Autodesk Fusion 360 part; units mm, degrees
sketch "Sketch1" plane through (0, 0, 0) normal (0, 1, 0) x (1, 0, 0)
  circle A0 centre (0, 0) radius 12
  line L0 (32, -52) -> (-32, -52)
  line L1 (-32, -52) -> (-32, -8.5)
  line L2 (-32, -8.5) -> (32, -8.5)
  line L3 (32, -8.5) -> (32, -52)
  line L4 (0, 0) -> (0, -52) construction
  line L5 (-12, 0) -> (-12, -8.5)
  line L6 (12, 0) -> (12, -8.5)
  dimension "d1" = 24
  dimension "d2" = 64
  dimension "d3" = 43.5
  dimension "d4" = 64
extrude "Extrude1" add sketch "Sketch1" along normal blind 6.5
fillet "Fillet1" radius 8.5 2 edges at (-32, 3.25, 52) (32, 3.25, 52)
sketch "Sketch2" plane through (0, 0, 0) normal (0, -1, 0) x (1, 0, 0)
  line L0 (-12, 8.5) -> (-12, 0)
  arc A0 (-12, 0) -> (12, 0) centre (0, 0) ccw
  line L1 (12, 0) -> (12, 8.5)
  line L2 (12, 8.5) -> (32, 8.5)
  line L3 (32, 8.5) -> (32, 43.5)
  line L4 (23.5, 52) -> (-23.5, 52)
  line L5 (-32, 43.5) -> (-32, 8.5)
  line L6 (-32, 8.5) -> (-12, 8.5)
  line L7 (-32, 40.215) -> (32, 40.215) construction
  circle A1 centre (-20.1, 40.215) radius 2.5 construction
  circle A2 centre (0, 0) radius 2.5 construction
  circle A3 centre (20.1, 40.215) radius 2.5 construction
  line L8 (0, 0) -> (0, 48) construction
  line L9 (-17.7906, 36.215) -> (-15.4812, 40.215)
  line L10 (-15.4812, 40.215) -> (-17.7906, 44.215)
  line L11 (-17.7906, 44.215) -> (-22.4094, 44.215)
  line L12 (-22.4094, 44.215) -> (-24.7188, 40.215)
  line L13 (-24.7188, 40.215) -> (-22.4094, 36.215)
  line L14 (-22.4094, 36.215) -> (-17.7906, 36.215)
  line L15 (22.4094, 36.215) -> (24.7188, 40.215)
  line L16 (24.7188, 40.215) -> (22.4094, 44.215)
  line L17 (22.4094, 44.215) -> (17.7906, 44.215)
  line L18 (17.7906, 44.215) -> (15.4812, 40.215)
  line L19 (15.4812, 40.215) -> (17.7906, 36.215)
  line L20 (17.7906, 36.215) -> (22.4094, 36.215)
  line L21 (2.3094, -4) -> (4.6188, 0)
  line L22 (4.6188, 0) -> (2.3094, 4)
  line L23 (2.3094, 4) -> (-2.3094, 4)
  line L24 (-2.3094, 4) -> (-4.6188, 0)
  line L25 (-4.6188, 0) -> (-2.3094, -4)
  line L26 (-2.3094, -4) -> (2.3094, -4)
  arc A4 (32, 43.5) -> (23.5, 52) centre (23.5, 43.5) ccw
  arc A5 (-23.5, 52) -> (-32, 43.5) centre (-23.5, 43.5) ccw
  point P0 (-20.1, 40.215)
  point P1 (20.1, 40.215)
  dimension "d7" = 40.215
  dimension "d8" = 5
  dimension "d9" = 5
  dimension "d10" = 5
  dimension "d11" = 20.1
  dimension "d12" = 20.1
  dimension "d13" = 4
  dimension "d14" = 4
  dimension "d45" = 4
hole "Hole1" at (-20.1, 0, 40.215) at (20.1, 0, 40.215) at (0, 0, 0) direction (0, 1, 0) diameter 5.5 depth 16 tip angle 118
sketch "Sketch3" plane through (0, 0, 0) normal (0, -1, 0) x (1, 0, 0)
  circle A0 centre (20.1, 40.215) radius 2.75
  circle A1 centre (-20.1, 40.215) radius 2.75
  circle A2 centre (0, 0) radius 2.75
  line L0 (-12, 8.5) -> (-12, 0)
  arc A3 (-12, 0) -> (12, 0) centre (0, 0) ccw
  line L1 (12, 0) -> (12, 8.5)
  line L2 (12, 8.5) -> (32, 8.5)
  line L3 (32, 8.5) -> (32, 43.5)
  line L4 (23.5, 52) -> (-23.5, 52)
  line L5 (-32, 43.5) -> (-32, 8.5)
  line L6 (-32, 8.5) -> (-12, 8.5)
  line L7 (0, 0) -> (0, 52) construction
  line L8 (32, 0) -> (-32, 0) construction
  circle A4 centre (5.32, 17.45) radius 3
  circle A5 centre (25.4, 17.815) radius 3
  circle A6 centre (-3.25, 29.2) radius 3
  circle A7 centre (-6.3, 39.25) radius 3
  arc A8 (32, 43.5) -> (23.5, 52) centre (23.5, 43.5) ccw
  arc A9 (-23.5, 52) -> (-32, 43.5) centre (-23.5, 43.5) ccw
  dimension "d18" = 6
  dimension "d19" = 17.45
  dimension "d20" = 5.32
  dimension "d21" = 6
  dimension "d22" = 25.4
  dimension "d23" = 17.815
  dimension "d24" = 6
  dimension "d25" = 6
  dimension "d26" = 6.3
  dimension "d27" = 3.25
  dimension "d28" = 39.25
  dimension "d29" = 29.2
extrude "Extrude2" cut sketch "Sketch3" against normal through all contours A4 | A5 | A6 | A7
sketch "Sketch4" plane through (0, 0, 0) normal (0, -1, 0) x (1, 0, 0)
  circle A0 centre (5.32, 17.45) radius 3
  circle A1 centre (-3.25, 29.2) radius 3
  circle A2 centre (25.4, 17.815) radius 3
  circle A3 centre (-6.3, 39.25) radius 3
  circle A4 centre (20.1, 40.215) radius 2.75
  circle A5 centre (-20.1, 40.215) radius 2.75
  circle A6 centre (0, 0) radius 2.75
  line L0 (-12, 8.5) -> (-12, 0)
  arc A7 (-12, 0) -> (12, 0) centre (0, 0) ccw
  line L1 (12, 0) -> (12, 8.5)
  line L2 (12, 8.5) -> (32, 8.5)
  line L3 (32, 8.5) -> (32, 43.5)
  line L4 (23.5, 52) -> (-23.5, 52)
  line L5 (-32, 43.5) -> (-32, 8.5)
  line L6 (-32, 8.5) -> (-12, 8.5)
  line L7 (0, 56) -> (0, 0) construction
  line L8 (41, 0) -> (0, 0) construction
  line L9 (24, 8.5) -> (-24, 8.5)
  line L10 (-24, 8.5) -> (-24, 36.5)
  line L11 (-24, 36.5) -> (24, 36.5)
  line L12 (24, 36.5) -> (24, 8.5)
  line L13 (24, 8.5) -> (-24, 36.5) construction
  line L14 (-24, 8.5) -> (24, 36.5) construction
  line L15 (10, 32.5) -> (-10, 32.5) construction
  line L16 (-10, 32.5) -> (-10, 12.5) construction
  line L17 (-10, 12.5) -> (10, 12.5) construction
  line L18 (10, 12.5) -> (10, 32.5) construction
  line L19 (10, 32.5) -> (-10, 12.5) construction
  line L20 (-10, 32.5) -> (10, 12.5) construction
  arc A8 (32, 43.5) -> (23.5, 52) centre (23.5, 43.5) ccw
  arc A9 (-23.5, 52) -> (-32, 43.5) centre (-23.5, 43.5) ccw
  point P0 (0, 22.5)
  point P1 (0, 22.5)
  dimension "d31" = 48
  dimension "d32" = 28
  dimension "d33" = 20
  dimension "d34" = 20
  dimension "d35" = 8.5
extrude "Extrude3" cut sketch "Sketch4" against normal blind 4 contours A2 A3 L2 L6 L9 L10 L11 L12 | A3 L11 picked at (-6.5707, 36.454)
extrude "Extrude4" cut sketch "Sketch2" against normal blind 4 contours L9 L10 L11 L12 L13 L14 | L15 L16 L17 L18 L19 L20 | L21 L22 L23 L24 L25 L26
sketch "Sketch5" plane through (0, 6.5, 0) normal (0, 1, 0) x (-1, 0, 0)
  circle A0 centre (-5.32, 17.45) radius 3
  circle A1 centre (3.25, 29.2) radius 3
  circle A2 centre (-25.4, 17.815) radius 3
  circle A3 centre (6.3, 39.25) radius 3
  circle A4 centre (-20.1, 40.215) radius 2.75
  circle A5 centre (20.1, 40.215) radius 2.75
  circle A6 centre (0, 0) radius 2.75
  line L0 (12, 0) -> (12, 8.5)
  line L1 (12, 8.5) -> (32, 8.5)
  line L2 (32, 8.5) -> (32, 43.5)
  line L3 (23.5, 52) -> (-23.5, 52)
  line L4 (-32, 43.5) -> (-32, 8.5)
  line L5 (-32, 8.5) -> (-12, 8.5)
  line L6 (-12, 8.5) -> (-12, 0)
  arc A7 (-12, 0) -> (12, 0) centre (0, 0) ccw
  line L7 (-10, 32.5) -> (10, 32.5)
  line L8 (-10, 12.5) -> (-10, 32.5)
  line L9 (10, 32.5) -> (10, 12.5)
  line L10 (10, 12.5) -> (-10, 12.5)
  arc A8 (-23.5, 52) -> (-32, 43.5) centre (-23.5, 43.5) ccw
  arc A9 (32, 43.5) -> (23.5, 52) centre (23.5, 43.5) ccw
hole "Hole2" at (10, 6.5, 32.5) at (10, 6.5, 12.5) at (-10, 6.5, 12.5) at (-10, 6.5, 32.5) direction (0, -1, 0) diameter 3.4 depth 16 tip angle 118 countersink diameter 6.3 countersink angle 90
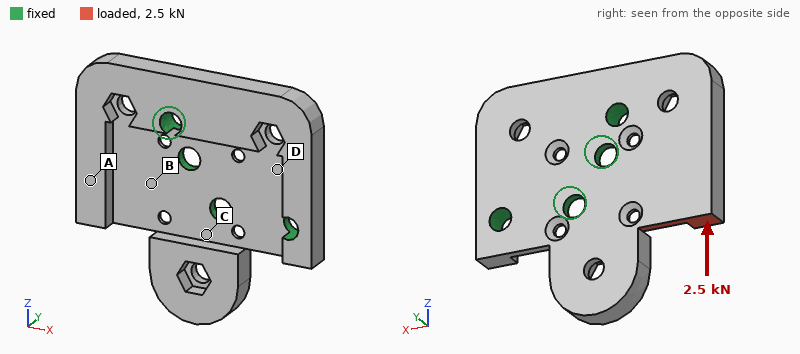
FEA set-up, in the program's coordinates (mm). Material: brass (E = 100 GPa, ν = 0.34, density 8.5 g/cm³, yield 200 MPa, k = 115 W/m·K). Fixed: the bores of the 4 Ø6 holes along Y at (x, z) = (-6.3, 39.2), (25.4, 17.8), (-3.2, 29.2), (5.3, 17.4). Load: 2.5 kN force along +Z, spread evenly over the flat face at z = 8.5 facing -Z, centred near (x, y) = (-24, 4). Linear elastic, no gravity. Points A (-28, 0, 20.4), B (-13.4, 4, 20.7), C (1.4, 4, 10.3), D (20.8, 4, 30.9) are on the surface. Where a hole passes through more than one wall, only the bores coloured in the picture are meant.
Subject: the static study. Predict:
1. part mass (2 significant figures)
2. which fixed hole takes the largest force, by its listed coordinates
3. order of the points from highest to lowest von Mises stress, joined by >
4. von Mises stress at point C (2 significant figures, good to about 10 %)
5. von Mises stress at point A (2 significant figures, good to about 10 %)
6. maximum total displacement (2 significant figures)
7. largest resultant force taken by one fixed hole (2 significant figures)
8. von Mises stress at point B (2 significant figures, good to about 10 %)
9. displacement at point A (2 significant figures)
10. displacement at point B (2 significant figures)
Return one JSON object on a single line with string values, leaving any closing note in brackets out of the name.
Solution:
{"part mass": "120 g", "which fixed hole takes the largest force, by its listed coordinates": "(-6.3, 39.2)", "order of the points from highest to lowest von Mises stress, joined by >": "B > A > C > D", "von Mises stress at point C": "18 MPa", "von Mises stress at point A": "31 MPa", "maximum total displacement": "43 µm", "largest resultant force taken by one fixed hole": "2.1 kN", "von Mises stress at point B": "53 MPa", "displacement at point A": "30 µm", "displacement at point B": "12 µm"}
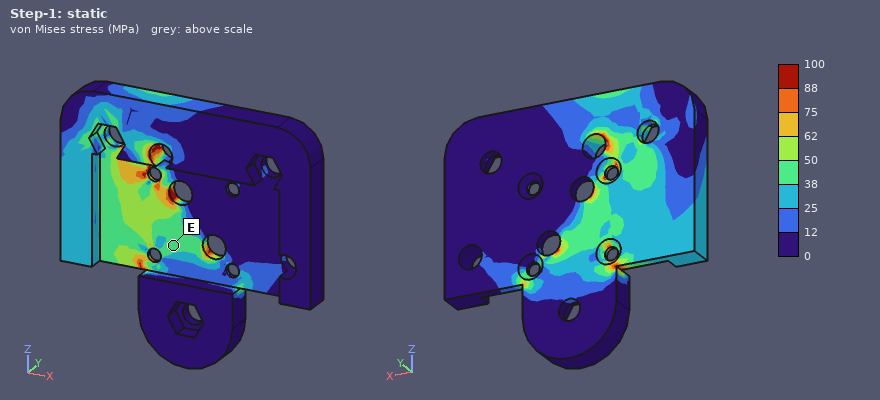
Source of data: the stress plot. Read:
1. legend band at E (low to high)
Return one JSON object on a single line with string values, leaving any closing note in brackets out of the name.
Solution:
{"legend band at E": "38 to 50 MPa"}
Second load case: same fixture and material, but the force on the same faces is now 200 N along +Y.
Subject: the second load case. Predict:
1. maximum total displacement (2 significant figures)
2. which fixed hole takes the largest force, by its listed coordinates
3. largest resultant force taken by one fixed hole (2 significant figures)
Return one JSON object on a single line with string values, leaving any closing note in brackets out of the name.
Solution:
{"maximum total displacement": "0.13 mm", "which fixed hole takes the largest force, by its listed coordinates": "(-3.2, 29.2)", "largest resultant force taken by one fixed hole": "160 N"}
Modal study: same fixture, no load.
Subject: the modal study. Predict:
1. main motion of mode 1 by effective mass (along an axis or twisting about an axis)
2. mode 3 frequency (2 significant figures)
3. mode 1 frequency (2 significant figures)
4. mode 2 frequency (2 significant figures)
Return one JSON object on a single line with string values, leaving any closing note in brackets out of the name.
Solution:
{"main motion of mode 1 by effective mass": "along Y", "mode 3 frequency": "4700 Hz", "mode 1 frequency": "1400 Hz", "mode 2 frequency": "2300 Hz"}
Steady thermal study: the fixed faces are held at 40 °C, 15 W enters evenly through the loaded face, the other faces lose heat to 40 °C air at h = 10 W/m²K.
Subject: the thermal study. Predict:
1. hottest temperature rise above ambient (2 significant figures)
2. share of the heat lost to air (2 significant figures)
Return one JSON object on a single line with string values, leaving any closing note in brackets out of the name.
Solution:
{"hottest temperature rise above ambient": "42 K", "share of the heat lost to air": "3.5 %"}
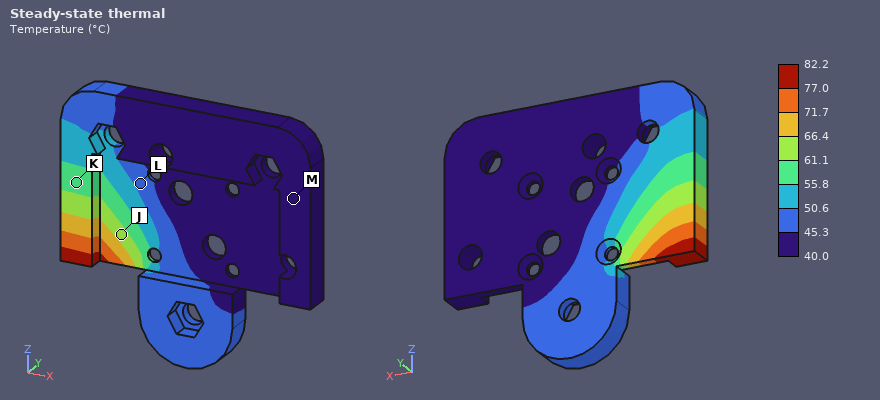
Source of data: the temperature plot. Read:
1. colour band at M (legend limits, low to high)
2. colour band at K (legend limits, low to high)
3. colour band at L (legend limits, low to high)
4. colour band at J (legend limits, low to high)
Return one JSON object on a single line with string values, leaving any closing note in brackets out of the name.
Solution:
{"colour band at M": "40.0 to 45.3 °C", "colour band at K": "55.8 to 61.1 °C", "colour band at L": "45.3 to 50.6 °C", "colour band at J": "61.1 to 66.4 °C"}
